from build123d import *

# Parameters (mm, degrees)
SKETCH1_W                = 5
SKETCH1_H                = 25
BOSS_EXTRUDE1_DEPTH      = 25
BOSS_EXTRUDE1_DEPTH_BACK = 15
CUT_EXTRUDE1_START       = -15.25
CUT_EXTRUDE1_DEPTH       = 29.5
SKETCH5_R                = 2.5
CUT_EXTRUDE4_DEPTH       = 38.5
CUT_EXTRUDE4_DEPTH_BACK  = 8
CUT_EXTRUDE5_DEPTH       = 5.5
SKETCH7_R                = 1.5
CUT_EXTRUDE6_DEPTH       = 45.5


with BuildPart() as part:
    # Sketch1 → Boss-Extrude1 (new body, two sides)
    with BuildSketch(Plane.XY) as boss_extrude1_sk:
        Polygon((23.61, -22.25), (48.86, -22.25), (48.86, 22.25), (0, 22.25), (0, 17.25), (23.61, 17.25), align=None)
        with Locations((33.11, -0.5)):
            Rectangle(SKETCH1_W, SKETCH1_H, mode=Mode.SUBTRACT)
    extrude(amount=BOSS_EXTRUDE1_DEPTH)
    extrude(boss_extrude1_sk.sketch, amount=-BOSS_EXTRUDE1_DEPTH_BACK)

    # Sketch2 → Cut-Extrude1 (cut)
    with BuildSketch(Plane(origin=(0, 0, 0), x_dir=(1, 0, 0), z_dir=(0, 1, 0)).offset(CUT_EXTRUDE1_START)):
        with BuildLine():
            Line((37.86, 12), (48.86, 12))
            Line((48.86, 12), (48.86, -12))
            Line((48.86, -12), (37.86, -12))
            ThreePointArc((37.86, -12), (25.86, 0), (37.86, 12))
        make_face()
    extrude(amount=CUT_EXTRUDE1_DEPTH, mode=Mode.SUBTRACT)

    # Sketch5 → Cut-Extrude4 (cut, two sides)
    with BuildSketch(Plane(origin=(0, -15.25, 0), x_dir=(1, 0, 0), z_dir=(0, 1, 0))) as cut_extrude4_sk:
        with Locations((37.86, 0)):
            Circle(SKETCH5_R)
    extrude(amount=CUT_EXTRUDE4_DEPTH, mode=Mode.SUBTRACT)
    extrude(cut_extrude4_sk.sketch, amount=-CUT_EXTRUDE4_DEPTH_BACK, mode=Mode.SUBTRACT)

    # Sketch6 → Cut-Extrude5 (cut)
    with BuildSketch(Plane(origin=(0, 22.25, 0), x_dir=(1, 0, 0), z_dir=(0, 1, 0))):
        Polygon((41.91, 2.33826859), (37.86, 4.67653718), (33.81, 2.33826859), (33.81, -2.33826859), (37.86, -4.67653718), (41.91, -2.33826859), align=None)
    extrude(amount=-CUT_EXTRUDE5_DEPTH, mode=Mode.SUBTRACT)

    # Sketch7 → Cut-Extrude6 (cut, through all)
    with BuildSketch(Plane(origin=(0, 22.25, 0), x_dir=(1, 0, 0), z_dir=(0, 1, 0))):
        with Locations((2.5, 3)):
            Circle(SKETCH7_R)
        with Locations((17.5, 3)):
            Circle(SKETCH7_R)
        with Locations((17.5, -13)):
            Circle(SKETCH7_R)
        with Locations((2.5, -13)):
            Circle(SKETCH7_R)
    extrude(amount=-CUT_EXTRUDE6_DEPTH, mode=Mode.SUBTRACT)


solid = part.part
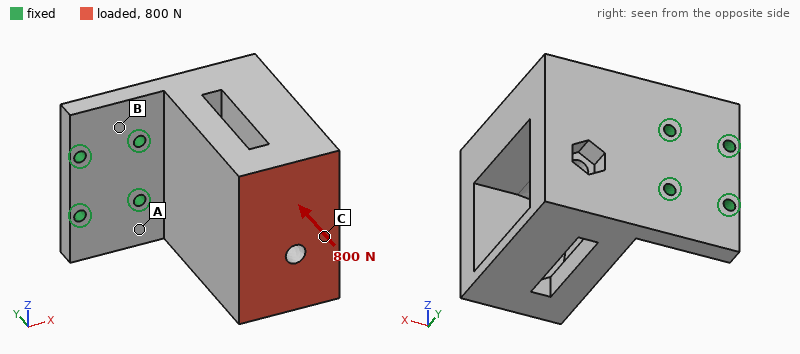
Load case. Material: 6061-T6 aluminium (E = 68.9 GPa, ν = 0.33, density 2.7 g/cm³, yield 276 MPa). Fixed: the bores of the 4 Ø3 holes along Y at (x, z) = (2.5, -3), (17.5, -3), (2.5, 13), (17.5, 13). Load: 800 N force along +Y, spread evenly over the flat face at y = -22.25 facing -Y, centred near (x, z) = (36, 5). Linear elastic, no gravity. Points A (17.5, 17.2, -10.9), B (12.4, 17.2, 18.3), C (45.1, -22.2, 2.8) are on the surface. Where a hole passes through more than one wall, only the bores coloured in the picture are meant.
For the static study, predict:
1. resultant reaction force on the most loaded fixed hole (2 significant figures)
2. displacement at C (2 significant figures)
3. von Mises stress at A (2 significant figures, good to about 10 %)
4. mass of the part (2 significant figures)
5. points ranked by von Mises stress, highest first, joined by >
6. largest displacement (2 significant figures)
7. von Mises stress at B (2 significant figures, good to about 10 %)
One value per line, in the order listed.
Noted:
590 N
0.20 mm
42 MPa
87 g
A > B > C
0.20 mm
20 MPa
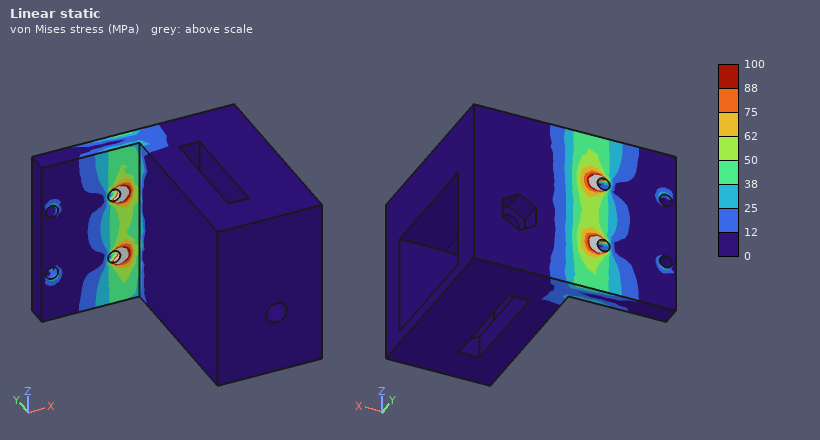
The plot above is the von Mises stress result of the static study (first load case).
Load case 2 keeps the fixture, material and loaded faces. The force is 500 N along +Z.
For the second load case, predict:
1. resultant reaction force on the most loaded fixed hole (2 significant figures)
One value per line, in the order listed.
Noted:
1.1 kN
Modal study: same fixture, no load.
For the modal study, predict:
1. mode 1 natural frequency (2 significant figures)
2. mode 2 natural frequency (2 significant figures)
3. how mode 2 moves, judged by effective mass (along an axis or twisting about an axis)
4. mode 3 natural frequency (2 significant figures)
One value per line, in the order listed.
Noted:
1100 Hz
2600 Hz
along Z
5600 Hz
